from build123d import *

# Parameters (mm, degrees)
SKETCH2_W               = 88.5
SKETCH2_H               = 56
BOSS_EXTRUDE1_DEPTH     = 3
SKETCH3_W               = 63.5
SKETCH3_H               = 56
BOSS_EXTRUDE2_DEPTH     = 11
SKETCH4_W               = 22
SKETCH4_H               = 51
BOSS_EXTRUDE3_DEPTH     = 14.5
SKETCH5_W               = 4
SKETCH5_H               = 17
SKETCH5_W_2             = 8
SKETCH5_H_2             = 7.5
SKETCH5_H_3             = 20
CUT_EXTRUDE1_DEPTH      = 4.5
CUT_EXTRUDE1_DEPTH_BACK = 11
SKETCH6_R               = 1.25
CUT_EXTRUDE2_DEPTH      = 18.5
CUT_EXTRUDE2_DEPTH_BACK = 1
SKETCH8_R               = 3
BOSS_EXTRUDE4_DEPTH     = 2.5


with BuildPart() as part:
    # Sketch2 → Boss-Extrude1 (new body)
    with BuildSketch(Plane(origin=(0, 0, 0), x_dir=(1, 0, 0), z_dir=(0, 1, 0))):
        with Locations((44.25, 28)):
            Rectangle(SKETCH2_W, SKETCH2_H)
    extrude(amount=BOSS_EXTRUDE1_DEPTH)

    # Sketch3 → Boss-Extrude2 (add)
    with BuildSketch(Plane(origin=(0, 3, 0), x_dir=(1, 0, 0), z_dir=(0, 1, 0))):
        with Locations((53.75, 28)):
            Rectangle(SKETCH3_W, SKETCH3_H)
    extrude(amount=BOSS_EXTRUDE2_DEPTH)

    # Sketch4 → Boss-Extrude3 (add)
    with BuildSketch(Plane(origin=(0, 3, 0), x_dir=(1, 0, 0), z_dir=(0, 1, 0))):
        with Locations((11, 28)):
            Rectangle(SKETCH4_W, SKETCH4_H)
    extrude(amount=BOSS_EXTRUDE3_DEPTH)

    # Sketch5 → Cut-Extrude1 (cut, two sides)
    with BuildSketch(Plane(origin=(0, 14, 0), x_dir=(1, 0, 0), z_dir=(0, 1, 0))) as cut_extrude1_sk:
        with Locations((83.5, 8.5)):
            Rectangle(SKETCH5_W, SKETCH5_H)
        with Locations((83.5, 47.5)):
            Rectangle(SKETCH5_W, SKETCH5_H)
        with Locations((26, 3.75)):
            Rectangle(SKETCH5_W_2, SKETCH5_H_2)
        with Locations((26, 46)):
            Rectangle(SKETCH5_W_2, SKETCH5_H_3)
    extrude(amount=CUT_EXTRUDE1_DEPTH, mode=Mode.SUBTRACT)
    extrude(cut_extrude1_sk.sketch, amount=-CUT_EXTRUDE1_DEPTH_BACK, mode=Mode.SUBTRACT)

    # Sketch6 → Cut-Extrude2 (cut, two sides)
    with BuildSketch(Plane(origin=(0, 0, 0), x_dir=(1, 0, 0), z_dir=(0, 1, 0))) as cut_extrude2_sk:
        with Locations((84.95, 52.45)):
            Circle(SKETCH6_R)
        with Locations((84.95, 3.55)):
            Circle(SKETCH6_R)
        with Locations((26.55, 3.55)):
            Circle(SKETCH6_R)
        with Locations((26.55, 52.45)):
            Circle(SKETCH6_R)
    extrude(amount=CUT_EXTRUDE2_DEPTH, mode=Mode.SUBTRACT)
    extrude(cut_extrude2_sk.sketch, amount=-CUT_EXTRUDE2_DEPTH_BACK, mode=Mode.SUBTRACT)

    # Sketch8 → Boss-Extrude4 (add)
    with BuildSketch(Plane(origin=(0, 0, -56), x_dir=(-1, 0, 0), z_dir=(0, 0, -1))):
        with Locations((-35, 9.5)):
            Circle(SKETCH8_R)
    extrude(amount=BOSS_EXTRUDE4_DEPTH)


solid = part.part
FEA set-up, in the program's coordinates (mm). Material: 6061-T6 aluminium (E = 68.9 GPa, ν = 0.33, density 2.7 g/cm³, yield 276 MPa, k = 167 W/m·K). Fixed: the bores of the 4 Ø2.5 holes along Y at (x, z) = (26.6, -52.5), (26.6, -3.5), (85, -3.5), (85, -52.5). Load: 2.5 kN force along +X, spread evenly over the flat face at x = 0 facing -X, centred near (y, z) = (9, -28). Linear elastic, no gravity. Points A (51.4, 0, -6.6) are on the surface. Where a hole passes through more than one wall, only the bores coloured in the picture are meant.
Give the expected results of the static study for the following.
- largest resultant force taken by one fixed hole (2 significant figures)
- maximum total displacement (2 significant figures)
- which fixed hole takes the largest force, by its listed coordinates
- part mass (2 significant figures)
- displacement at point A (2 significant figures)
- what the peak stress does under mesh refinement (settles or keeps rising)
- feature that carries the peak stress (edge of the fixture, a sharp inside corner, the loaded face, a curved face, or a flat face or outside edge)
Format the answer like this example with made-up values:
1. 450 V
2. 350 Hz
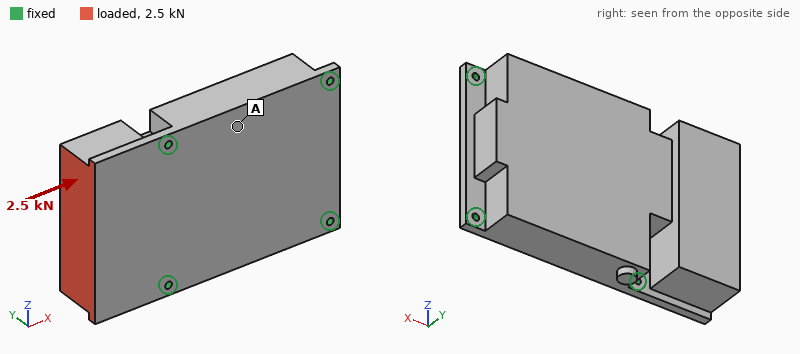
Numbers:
1. 850 N
2. 21 µm
3. (26.6, -52.5)
4. 180 g
5. 3.4 µm
6. keeps rising
7. edge of the fixture
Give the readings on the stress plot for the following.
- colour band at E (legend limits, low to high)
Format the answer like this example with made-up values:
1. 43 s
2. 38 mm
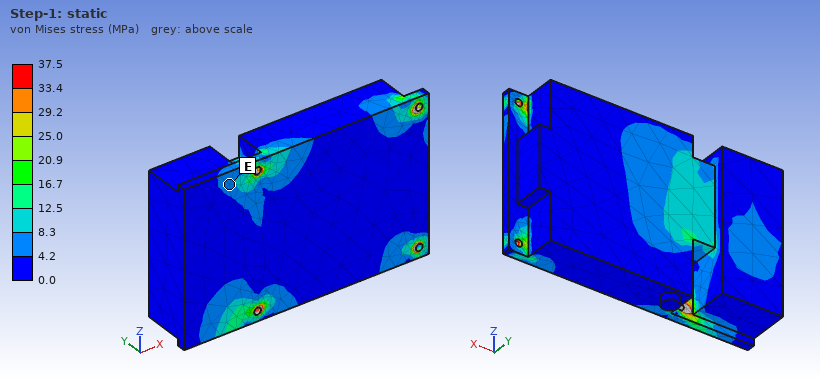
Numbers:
1. 4.2 to 8.3 MPa
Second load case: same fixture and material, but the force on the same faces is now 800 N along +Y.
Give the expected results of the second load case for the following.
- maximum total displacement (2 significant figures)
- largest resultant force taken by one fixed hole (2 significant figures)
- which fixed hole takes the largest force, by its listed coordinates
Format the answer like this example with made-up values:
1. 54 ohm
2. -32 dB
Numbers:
1. 37 µm
2. 770 N
3. (26.6, -3.5)
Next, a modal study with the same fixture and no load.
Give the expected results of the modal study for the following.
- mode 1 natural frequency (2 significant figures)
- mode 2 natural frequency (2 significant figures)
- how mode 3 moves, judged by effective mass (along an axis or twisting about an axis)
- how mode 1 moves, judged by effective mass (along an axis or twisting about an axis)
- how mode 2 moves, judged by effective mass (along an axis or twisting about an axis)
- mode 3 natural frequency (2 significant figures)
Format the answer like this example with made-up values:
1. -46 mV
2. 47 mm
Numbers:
1. 4600 Hz
2. 6600 Hz
3. along Z
4. along Y
5. along Y
6. 8800 Hz
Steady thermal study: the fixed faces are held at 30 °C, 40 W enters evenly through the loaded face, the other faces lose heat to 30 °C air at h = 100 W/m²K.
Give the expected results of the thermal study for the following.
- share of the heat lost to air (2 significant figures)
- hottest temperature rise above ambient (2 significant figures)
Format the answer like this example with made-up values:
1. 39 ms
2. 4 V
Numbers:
1. 26 %
2. 17 K
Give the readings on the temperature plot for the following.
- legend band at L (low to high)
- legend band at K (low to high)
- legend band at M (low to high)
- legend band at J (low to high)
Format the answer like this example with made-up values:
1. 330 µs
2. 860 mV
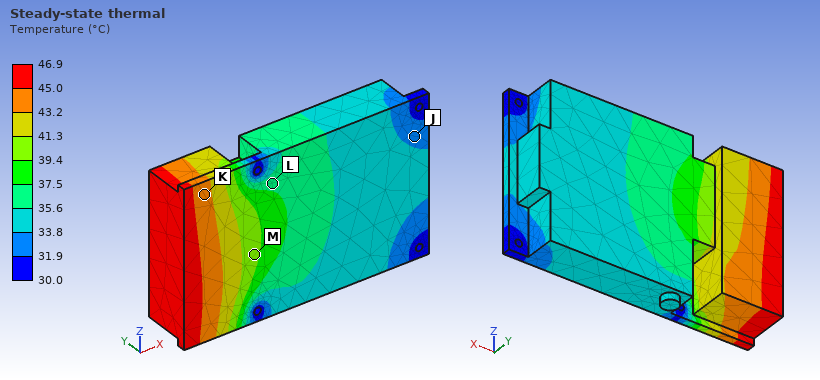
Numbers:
1. 35.6 to 37.5 °C
2. 43.2 to 45.0 °C
3. 39.4 to 41.3 °C
4. 31.9 to 33.8 °C
